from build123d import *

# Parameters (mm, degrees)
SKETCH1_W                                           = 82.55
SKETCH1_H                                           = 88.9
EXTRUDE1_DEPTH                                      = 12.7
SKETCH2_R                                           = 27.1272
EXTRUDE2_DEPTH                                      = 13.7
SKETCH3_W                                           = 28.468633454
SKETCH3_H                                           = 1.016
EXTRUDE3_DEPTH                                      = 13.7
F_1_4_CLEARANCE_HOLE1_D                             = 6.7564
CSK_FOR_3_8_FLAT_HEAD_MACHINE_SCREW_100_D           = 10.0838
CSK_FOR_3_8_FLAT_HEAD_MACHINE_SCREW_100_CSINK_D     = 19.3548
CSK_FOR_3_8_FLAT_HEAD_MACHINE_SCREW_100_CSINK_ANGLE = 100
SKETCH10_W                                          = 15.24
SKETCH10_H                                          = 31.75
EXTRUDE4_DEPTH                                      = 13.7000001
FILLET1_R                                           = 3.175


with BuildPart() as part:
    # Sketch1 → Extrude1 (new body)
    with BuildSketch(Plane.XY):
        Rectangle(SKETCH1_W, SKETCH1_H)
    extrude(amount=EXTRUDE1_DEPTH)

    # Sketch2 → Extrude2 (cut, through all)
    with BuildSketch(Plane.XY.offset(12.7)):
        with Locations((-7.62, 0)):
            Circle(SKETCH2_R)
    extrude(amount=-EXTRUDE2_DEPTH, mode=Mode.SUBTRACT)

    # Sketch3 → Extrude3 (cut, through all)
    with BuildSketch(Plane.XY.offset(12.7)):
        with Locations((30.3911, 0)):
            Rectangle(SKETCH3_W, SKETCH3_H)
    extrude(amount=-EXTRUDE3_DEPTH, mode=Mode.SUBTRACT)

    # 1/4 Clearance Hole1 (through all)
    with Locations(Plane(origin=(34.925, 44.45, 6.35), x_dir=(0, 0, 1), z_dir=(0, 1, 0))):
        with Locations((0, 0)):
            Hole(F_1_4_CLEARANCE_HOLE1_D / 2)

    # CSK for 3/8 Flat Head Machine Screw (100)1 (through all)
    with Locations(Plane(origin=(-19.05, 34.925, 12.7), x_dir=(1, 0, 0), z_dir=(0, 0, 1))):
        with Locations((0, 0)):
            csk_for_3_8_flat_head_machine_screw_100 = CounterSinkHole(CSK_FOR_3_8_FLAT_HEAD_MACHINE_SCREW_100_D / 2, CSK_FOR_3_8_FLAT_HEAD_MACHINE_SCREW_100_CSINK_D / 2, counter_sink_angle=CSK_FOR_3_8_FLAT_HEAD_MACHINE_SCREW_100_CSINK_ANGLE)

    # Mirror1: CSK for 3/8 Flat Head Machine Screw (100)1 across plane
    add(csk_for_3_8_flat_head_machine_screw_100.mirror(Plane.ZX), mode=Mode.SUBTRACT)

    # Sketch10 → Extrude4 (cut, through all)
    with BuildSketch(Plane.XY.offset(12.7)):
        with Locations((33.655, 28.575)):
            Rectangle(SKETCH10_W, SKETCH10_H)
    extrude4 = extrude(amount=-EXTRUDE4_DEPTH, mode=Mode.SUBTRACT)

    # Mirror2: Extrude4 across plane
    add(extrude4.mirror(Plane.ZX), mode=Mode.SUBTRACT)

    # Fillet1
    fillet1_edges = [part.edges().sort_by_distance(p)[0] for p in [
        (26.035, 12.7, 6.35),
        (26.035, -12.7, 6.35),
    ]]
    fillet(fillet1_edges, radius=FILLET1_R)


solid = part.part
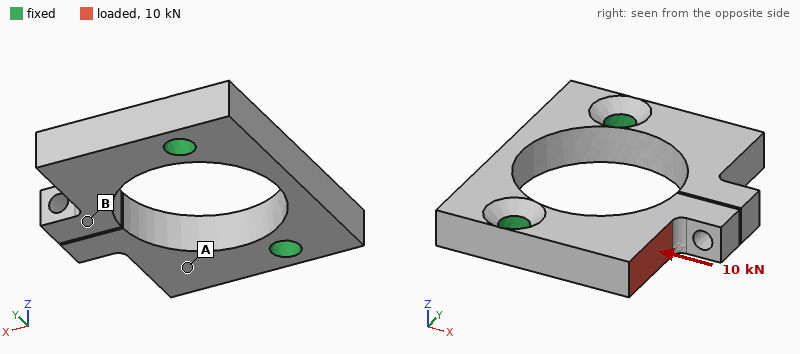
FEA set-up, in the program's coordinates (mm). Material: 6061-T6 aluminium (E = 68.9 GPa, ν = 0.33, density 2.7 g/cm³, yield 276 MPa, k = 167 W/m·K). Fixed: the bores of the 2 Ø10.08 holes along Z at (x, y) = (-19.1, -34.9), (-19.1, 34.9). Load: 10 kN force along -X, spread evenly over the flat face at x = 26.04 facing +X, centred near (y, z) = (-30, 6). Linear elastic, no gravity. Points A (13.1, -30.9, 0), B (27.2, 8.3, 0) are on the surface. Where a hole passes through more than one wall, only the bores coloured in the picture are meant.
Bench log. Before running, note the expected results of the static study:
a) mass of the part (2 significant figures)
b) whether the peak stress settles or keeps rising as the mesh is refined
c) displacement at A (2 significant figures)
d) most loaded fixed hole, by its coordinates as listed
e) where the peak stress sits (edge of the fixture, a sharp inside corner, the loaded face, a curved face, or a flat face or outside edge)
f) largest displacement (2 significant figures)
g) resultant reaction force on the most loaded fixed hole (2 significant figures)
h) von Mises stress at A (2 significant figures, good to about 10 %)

130 g
keeps rising
0.081 mm
(-19.1, -34.9)
edge of the fixture
0.24 mm
9.9 kN
43 MPa
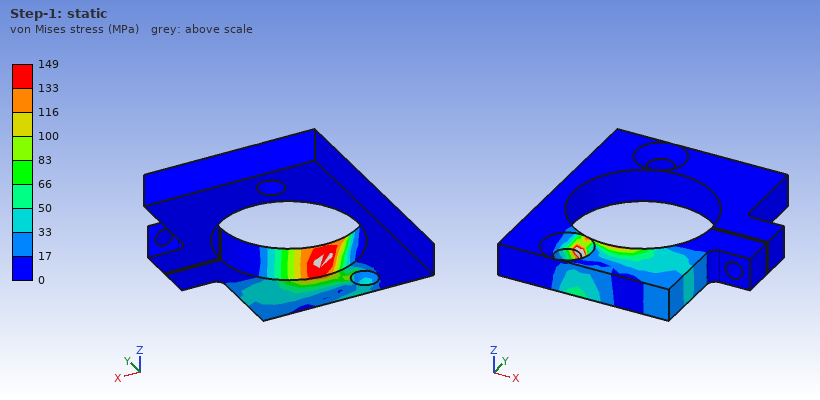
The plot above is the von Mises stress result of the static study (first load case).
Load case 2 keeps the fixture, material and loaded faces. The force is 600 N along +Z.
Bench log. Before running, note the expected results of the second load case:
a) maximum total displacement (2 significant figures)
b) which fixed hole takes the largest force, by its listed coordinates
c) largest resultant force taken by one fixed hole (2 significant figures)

0.16 mm
(-19.1, -34.9)
610 N
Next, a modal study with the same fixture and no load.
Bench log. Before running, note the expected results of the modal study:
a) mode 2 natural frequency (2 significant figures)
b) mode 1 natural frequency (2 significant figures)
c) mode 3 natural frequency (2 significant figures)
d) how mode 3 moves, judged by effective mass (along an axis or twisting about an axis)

2300 Hz
2300 Hz
3100 Hz
along Y
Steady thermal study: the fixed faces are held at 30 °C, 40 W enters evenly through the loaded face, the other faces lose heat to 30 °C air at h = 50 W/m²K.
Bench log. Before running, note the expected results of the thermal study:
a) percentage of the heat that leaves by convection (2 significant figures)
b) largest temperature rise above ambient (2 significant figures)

14 %
35 K
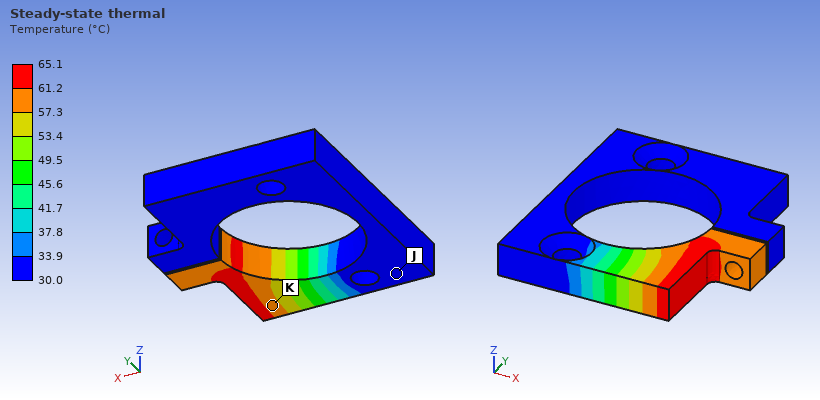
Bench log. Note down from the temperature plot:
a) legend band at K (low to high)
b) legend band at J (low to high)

57.3 to 61.2 °C
30.0 to 33.9 °C
